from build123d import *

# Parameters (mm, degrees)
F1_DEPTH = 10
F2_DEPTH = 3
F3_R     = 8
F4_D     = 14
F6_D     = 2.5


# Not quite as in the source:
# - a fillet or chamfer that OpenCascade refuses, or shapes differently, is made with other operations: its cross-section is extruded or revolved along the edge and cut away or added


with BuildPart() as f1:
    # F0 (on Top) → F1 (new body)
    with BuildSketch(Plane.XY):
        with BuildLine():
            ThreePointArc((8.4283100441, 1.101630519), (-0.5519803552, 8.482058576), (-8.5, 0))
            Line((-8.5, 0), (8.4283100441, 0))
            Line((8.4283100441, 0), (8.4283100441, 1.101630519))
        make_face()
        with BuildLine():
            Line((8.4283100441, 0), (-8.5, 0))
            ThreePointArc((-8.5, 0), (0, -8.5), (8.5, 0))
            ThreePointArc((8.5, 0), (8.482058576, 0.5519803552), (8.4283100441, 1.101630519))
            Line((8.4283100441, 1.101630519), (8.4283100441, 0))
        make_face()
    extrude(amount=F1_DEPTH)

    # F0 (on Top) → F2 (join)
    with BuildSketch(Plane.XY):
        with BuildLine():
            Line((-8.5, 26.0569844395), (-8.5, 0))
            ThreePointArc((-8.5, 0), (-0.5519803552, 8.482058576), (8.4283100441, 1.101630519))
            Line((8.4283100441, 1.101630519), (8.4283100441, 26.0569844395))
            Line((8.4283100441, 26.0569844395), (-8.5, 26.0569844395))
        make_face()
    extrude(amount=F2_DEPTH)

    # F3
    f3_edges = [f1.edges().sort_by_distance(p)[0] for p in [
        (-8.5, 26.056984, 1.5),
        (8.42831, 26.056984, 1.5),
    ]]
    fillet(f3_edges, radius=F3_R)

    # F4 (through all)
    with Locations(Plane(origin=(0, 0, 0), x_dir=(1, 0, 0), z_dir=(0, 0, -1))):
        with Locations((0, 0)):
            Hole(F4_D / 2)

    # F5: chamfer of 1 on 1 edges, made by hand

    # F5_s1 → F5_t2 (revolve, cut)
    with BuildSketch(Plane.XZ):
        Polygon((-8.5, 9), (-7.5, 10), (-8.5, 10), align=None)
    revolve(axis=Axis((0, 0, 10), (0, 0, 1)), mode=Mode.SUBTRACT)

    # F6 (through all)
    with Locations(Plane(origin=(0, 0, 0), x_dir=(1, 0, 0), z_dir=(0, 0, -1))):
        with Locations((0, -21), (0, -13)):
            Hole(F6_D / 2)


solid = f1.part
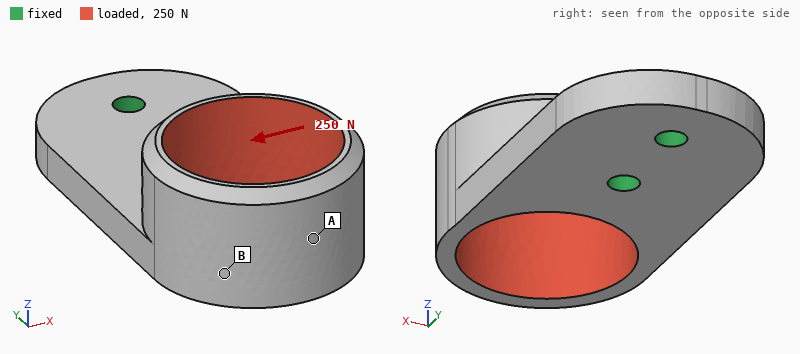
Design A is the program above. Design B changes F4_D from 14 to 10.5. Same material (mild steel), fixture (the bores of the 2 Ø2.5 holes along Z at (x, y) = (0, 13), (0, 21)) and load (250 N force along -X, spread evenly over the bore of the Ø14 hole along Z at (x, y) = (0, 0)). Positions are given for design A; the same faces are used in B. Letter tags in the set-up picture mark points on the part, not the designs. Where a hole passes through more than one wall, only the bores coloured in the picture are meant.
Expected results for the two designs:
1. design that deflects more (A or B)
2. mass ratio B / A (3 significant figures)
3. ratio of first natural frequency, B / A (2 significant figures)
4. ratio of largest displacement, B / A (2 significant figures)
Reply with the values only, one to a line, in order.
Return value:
A
1.43
0.84
0.44
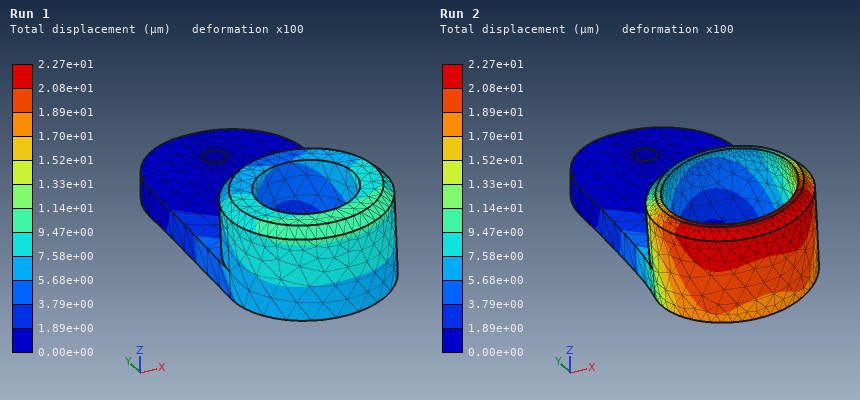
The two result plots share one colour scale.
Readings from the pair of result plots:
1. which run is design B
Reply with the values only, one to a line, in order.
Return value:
Run 1
